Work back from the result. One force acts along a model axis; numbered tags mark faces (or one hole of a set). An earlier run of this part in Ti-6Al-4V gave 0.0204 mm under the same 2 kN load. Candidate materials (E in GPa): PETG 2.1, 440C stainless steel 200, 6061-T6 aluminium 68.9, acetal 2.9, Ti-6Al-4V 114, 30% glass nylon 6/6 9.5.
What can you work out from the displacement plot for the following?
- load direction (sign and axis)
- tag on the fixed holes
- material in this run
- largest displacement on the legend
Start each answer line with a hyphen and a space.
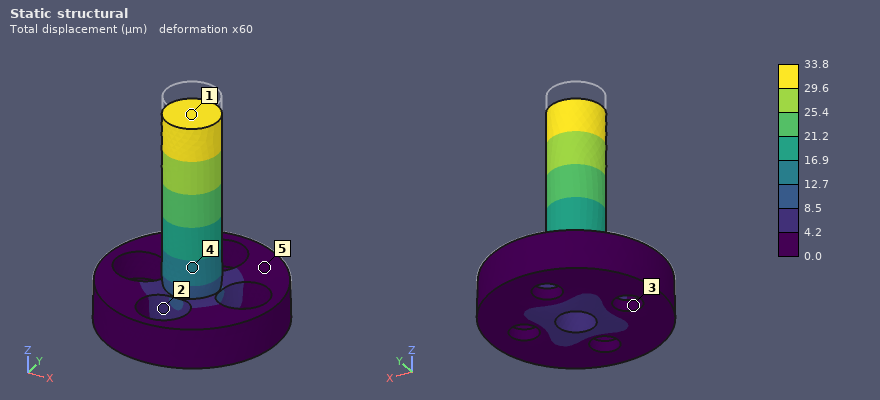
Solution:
- -Z
- 3
- 6061-T6 aluminium
- 33.8 µm
